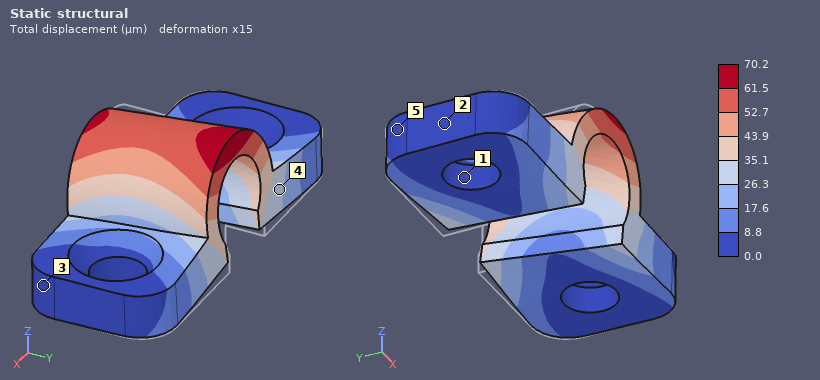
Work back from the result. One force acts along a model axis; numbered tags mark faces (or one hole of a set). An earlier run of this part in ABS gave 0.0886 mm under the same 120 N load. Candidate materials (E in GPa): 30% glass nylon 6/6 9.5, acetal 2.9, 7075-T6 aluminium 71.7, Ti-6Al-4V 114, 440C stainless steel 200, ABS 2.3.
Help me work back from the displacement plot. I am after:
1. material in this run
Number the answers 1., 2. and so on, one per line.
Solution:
1. acetal
